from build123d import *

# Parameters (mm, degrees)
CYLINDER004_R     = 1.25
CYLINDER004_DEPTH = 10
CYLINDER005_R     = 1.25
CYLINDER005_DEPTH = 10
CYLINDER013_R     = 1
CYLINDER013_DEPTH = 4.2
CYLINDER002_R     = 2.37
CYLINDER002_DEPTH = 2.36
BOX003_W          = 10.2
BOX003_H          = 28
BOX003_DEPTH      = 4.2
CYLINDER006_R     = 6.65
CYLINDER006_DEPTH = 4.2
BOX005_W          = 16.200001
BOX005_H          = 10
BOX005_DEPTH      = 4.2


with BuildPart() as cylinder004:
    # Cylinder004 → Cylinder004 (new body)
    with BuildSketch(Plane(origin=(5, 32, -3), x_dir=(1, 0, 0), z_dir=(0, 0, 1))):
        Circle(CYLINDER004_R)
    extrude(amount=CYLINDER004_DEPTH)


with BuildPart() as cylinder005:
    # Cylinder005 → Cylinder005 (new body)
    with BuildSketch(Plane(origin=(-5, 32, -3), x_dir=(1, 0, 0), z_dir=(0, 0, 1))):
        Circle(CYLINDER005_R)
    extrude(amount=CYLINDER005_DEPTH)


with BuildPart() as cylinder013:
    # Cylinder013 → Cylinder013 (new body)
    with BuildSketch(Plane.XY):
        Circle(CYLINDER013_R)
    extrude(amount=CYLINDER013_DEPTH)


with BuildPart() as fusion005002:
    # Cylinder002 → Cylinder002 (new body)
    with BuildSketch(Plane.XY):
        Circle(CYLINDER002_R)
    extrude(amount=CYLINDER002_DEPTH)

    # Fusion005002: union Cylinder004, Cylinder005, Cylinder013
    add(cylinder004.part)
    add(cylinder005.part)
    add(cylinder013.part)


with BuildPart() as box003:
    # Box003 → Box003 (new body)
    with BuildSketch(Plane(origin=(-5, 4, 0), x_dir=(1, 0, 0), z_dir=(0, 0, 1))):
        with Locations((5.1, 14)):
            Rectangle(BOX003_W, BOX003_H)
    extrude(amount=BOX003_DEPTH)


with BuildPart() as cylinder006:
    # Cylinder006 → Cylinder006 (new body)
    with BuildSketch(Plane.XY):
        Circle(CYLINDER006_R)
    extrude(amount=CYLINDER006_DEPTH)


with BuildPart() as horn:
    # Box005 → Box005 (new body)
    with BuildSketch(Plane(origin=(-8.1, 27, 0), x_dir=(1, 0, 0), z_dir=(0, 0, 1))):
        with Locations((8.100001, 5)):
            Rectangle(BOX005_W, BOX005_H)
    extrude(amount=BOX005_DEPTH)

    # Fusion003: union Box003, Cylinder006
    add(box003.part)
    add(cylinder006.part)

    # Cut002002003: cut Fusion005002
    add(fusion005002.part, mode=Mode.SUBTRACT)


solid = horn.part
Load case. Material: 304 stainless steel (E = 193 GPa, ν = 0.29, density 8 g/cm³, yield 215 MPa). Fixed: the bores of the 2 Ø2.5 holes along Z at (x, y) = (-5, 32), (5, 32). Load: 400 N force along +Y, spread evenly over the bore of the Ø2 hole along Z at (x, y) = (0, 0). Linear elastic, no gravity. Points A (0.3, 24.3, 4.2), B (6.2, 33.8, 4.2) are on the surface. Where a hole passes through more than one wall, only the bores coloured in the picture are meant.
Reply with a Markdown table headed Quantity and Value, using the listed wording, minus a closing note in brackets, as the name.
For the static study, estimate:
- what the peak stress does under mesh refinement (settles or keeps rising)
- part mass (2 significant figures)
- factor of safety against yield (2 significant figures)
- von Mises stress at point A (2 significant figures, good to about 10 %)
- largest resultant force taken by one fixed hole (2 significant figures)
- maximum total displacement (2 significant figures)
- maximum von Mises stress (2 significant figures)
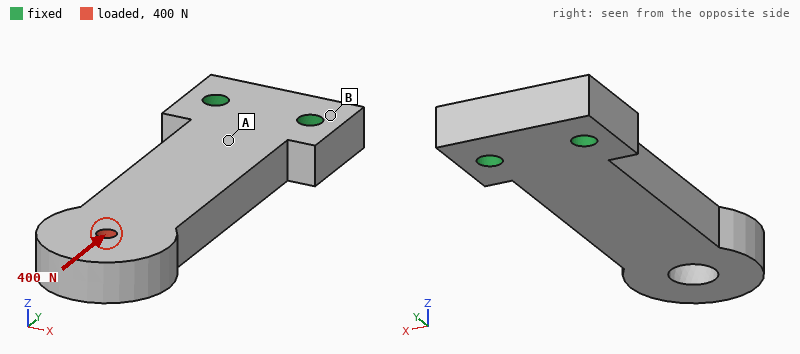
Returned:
| Quantity | Value |
|---|---|
| what the peak stress does under mesh refinement | settles |
| part mass | 17 g |
| factor of safety against yield | 3.1 |
| von Mises stress at point A | 23 MPa |
| largest resultant force taken by one fixed hole | 210 N |
| maximum total displacement | 27 µm |
| maximum von Mises stress | 68 MPa |
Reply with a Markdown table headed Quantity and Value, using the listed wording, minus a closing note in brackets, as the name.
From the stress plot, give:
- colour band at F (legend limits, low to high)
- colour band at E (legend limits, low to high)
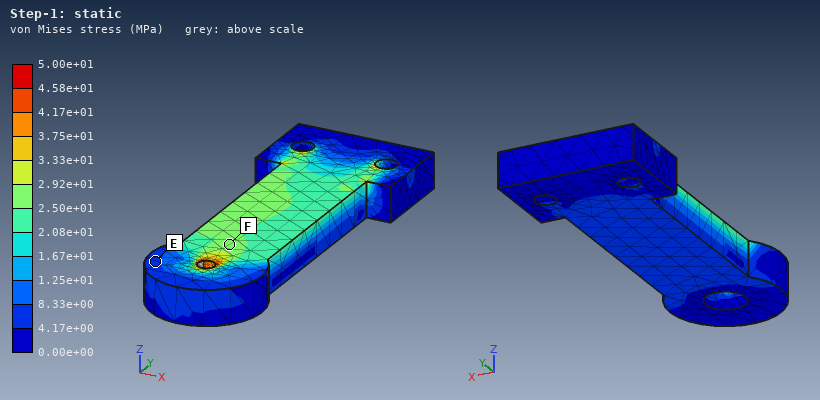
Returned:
| Quantity | Value |
|---|---|
| colour band at F | 2.50e+01 to 2.92e+01 MPa |
| colour band at E | 4.17e+00 to 8.33e+00 MPa |
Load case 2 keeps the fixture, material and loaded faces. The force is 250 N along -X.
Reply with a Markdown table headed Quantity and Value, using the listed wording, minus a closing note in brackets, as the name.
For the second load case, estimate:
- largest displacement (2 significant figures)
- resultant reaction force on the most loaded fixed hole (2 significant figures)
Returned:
| Quantity | Value |
|---|---|
| largest displacement | 44 µm |
| resultant reaction force on the most loaded fixed hole | 770 N |
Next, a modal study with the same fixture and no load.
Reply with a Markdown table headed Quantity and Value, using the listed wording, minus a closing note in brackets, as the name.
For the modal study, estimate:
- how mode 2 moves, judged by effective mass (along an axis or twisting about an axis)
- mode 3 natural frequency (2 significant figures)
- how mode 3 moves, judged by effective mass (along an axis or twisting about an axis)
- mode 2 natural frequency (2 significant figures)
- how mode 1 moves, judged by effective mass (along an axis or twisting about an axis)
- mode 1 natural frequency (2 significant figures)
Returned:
| Quantity | Value |
|---|---|
| how mode 2 moves, judged by effective mass | along X |
| mode 3 natural frequency | 13 kHz |
| how mode 3 moves, judged by effective mass | twisting about Y |
| mode 2 natural frequency | 5900 Hz |
| how mode 1 moves, judged by effective mass | along Z |
| mode 1 natural frequency | 2400 Hz |
